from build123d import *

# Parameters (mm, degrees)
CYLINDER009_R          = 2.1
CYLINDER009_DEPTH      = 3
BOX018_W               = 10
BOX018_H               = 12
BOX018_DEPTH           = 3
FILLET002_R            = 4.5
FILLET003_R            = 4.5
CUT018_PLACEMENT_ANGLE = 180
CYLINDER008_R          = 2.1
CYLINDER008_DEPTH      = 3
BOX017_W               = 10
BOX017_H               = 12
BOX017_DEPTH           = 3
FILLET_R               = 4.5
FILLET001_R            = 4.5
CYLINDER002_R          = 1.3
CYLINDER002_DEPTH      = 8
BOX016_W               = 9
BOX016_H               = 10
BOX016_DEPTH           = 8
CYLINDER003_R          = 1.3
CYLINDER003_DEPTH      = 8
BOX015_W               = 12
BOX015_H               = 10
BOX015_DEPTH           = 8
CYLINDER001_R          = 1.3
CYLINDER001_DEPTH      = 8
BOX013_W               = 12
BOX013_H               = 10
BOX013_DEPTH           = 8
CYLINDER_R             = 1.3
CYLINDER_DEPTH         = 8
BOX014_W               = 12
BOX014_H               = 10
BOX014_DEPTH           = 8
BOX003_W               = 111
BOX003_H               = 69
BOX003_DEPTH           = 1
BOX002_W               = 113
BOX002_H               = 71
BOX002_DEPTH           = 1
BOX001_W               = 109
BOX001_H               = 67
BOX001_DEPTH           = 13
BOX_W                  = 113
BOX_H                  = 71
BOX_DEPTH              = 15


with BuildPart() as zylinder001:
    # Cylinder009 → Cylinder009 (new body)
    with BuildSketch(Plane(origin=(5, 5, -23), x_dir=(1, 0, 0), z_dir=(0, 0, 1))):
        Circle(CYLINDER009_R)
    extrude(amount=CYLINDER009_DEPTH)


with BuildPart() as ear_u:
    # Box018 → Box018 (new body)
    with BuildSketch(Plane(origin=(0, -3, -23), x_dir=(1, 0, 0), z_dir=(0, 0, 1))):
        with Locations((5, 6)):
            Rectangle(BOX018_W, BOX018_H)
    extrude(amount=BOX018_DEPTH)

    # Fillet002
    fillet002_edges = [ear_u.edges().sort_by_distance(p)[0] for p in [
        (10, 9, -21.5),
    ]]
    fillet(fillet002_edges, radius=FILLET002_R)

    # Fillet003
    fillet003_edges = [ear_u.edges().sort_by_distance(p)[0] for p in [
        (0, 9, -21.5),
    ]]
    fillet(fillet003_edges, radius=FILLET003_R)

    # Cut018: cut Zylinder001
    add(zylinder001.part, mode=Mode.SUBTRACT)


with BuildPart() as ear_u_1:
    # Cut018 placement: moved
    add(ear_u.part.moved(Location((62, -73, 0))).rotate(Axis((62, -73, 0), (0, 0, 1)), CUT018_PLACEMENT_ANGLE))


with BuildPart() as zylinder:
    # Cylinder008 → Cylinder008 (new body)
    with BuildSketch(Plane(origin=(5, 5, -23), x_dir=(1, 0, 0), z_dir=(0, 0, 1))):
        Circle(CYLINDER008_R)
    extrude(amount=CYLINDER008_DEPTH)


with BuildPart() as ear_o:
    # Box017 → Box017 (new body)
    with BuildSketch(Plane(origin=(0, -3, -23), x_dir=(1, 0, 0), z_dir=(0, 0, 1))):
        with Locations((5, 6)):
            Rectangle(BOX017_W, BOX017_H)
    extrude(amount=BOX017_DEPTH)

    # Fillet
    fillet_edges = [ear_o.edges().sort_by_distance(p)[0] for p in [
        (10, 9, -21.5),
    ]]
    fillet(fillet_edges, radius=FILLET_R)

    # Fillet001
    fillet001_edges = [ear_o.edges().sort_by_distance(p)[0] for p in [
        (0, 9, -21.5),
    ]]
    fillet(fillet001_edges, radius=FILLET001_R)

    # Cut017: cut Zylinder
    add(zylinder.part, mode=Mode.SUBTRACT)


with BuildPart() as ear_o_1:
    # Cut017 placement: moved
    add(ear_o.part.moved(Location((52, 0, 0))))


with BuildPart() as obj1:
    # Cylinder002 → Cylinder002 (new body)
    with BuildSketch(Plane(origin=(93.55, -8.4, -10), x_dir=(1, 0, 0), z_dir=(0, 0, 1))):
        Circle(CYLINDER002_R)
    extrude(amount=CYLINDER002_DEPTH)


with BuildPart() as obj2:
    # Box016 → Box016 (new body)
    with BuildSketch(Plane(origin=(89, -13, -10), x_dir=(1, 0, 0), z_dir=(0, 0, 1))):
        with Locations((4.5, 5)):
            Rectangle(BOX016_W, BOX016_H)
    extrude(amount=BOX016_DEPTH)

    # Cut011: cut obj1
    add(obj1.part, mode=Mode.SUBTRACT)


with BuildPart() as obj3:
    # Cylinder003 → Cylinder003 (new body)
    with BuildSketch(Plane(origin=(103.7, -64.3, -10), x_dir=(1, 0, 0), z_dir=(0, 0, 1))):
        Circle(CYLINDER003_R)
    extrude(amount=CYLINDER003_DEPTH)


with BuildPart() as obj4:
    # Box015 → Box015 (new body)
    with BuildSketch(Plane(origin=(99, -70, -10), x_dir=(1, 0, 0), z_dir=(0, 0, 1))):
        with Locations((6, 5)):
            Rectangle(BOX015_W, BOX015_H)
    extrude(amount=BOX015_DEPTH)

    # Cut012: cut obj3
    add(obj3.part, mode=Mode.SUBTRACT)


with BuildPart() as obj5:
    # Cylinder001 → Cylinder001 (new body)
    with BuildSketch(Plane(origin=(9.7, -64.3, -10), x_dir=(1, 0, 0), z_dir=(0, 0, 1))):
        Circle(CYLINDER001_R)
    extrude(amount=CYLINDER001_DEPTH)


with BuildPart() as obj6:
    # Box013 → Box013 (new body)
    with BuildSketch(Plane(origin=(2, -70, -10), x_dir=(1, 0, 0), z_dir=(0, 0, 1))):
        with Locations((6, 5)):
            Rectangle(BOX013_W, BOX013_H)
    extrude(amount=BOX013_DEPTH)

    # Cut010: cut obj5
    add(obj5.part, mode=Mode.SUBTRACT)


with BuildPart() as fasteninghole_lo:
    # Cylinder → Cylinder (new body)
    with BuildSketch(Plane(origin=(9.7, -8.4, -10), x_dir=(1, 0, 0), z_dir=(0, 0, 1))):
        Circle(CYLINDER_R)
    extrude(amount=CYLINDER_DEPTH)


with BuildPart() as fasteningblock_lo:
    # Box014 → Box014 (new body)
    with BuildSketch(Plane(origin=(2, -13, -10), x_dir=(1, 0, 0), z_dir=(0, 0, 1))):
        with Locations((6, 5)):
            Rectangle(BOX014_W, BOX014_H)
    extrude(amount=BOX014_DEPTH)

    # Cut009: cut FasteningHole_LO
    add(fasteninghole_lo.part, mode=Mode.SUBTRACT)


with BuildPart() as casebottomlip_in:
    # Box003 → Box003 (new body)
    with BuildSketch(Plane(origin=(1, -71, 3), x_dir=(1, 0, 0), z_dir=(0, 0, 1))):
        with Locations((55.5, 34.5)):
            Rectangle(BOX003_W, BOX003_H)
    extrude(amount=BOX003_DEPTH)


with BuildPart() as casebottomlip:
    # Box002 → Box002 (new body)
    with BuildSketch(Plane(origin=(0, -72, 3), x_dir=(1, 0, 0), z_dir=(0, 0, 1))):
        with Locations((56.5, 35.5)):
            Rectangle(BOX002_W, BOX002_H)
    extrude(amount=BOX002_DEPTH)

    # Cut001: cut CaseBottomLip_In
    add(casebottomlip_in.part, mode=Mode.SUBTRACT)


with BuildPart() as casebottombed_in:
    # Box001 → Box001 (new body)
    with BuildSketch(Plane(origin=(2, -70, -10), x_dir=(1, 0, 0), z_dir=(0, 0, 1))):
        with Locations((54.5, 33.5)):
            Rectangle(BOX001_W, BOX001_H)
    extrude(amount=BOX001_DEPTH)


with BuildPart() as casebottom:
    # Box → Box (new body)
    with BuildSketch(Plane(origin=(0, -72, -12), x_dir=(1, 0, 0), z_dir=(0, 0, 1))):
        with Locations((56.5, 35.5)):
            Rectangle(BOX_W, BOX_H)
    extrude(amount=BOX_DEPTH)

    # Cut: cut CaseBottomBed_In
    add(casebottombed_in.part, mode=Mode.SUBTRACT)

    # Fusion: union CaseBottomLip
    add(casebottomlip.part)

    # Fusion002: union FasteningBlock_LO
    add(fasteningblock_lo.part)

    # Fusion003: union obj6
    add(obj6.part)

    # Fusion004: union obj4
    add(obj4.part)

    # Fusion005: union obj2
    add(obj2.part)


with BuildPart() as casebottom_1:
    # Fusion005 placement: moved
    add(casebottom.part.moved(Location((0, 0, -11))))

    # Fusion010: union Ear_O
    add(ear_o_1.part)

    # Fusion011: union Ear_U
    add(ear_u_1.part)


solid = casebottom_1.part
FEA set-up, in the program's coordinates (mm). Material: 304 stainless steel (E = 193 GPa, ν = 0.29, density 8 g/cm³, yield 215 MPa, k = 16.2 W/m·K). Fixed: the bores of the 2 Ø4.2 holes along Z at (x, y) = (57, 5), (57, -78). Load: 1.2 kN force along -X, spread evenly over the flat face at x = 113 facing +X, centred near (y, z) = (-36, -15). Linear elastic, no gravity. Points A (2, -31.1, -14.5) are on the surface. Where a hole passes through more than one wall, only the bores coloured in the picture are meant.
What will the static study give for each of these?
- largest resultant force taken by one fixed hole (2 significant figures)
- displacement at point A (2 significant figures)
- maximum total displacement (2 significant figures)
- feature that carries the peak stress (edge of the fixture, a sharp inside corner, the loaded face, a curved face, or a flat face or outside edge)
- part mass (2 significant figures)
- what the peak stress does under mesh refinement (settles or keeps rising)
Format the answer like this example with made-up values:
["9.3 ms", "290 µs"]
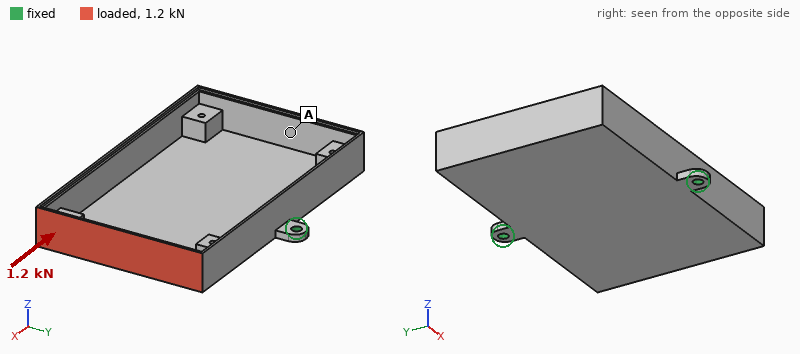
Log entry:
["600 N", "0.16 mm", "0.23 mm", "edge of the fixture", "240 g", "keeps rising"]
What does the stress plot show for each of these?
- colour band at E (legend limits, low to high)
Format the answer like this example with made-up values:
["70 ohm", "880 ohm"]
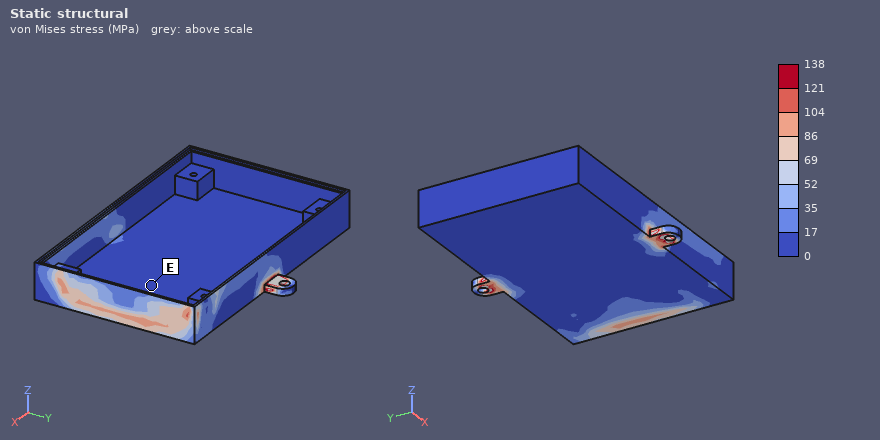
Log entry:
["0 to 17 MPa"]
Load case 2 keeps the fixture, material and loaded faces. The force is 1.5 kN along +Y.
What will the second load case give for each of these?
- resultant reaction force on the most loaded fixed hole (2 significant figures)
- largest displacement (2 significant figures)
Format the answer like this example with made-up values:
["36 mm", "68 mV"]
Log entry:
["1.3 kN", "0.23 mm"]
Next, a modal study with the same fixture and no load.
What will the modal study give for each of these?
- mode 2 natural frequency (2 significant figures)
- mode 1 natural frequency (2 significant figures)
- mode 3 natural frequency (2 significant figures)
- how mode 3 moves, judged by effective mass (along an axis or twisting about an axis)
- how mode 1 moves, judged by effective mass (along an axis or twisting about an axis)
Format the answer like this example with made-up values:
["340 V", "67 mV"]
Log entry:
["920 Hz", "430 Hz", "1500 Hz", "along Z", "twisting about Y"]
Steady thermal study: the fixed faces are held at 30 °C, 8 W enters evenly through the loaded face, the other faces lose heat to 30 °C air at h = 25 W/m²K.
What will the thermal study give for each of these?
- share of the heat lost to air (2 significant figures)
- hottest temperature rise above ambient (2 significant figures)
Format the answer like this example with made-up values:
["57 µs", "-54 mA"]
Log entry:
["94 %", "66 K"]
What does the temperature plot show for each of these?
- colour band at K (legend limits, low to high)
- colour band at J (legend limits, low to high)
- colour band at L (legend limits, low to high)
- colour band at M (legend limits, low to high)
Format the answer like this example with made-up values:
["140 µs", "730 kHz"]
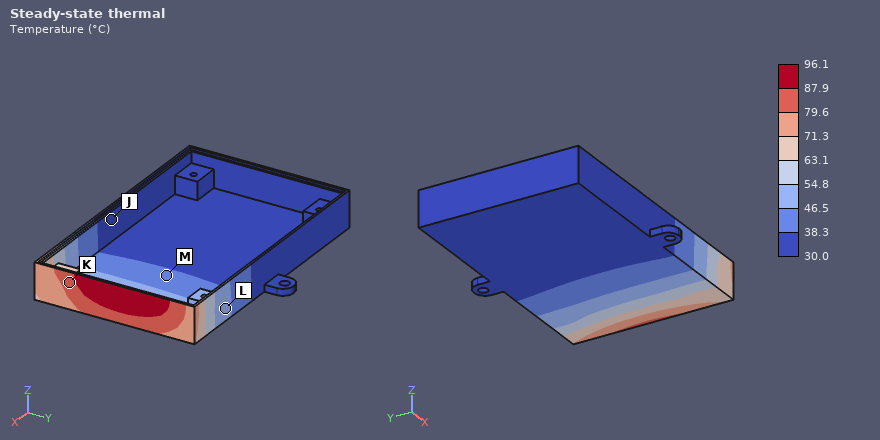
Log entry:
["79.6 to 87.9 °C", "30.0 to 38.3 °C", "46.5 to 54.8 °C", "38.3 to 46.5 °C"]
